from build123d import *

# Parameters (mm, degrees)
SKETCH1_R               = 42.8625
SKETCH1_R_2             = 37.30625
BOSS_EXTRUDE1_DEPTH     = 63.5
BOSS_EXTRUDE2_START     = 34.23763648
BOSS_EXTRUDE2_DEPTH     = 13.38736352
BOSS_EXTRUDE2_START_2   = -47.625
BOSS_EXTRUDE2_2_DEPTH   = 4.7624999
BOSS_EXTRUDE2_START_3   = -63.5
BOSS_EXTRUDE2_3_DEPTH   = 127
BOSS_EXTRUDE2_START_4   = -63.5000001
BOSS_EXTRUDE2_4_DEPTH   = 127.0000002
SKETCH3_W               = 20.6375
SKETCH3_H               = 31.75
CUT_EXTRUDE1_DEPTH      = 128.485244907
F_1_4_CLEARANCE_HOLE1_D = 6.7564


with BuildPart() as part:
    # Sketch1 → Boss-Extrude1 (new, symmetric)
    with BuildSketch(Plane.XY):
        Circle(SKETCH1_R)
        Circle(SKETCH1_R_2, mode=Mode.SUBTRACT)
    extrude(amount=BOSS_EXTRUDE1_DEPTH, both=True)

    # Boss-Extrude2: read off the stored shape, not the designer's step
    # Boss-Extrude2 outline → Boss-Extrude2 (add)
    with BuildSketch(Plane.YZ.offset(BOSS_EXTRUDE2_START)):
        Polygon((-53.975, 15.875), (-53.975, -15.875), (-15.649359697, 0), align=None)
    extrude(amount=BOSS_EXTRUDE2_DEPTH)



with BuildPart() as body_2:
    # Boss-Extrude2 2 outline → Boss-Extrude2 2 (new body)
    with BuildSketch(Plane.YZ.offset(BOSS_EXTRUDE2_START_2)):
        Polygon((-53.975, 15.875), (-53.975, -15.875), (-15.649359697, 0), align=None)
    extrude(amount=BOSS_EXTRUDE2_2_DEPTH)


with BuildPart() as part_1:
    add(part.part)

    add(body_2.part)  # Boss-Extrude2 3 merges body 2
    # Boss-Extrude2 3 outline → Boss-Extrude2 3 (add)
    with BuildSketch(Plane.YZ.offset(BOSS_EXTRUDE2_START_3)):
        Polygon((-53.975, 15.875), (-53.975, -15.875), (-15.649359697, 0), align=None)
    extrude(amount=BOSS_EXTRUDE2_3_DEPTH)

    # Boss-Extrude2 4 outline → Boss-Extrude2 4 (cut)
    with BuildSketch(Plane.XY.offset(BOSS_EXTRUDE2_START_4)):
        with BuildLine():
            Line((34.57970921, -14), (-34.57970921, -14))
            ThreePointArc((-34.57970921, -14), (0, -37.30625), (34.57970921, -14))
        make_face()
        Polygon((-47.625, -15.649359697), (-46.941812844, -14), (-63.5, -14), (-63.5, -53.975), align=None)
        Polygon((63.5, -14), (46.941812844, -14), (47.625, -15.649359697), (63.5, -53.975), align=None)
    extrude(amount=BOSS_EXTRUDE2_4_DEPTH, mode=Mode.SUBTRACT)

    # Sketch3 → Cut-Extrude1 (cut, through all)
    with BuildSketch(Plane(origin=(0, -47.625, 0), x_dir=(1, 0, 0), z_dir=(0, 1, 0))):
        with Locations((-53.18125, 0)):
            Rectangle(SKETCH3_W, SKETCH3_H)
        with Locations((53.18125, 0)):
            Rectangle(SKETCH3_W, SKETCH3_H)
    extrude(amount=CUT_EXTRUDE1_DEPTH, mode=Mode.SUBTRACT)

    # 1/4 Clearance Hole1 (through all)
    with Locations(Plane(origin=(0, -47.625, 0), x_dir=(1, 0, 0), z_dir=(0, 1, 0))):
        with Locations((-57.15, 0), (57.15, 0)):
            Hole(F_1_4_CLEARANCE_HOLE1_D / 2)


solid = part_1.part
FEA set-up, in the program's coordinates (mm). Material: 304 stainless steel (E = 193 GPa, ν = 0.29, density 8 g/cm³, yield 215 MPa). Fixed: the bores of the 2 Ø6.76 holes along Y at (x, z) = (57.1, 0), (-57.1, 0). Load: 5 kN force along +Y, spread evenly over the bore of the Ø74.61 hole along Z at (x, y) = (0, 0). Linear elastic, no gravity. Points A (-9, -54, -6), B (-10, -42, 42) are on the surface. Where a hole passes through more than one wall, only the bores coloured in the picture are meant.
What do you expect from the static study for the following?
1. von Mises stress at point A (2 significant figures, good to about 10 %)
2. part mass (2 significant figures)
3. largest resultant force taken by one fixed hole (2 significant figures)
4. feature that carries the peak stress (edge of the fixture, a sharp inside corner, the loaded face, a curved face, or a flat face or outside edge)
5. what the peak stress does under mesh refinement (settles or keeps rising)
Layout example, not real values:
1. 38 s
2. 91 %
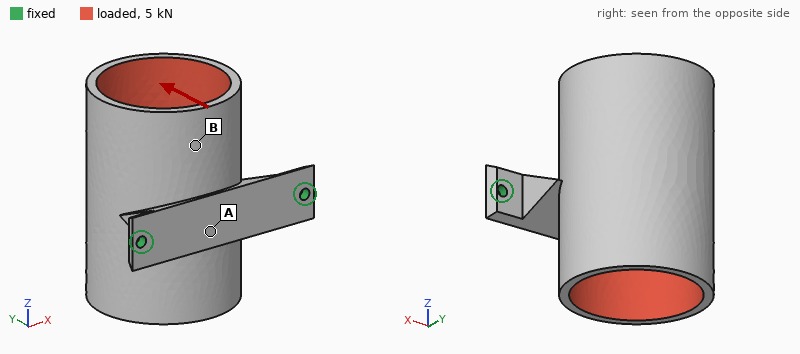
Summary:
1. 11 MPa
2. 1.8 kg
3. 3.0 kN
4. edge of the fixture
5. keeps rising
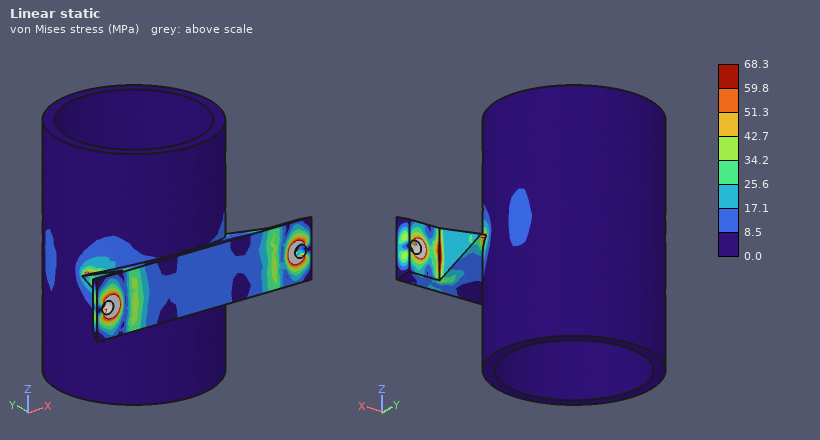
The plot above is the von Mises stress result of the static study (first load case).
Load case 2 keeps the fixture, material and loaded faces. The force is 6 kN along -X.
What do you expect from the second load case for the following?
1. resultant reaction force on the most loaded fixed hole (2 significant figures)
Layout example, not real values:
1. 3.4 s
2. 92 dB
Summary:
1. 4.3 kN
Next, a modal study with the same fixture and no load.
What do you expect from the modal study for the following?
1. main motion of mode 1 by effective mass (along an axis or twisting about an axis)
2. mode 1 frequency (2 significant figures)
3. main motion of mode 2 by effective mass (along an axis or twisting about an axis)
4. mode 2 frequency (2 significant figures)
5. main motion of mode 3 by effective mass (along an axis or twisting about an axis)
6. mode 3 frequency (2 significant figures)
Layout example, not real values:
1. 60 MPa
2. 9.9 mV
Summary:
1. along Z
2. 290 Hz
3. along X
4. 960 Hz
5. twisting about Y
6. 1500 Hz
